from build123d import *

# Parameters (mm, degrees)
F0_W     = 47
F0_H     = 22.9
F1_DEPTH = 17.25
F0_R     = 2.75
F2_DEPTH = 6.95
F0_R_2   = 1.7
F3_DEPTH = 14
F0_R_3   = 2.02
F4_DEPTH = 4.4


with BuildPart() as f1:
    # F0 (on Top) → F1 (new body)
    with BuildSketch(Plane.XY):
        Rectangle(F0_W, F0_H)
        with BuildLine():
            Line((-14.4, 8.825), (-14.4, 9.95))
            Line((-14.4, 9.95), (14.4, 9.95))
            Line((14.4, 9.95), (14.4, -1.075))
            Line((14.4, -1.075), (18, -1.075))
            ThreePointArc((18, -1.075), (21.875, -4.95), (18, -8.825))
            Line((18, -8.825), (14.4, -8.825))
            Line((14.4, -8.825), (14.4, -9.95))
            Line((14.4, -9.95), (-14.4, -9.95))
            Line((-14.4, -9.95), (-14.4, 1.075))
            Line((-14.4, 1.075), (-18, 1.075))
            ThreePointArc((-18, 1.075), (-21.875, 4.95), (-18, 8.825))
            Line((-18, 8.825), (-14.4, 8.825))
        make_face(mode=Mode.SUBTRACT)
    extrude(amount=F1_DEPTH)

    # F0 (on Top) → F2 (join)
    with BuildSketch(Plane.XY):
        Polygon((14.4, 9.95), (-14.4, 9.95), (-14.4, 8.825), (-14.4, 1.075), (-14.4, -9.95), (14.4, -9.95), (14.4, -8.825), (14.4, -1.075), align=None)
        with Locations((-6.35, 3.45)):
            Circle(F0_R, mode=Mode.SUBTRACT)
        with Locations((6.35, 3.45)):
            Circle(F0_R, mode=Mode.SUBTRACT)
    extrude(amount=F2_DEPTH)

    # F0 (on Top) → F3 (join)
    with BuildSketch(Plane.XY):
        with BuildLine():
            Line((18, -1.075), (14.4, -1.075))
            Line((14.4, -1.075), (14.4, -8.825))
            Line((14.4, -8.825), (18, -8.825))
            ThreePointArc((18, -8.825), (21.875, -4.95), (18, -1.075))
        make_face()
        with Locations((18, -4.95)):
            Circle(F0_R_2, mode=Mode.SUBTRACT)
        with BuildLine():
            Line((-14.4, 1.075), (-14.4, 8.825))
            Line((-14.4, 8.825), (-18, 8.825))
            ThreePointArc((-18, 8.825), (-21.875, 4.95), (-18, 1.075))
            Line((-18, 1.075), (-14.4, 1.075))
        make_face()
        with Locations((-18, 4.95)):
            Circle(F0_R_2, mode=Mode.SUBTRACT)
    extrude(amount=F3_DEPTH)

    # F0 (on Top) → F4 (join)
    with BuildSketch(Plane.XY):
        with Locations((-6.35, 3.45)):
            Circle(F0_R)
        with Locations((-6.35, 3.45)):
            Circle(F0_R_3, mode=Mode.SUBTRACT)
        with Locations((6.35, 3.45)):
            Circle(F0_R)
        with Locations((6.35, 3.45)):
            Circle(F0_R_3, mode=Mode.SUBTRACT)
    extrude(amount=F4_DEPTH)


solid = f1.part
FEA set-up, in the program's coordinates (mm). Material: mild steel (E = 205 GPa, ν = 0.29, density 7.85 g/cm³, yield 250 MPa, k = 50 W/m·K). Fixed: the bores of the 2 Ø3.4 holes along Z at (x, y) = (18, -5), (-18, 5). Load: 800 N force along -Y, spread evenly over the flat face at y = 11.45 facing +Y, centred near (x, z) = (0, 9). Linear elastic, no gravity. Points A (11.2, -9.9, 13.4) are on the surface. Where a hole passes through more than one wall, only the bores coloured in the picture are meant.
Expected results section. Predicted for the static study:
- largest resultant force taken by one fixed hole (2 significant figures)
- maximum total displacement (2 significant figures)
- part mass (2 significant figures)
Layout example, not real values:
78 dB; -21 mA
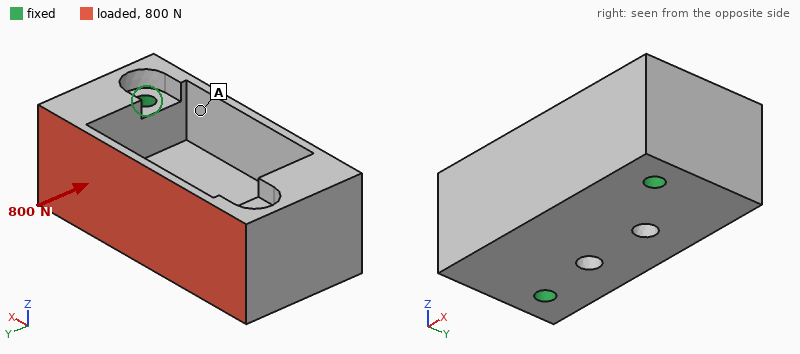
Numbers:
410 N; 17 µm; 93 g
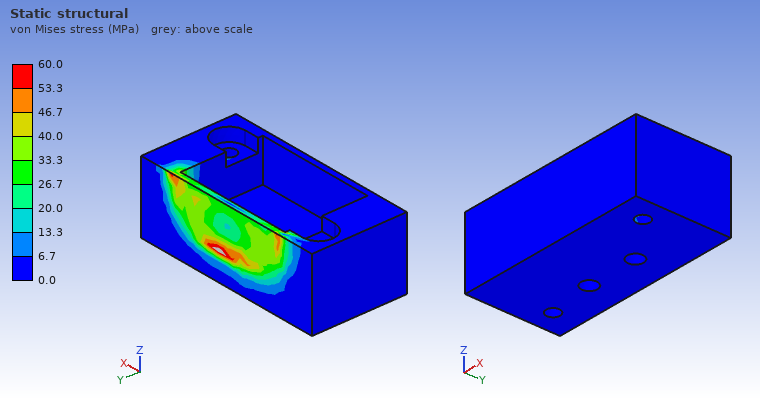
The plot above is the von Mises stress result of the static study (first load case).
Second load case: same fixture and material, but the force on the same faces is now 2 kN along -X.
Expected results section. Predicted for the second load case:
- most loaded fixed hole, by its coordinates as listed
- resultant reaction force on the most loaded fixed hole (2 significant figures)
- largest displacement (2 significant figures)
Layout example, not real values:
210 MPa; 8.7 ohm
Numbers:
(-18, 5); 1.4 kN; 3.0 µm
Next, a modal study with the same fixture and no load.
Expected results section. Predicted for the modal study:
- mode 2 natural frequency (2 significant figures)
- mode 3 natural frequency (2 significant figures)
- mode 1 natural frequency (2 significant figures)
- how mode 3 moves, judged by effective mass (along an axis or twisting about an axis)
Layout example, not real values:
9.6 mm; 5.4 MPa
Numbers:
16 kHz; 22 kHz; 15 kHz; along Z
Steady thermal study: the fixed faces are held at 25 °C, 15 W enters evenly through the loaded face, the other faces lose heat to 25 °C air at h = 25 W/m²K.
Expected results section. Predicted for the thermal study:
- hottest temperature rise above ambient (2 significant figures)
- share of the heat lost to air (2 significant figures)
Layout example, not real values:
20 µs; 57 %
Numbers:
22 K; 3.6 %
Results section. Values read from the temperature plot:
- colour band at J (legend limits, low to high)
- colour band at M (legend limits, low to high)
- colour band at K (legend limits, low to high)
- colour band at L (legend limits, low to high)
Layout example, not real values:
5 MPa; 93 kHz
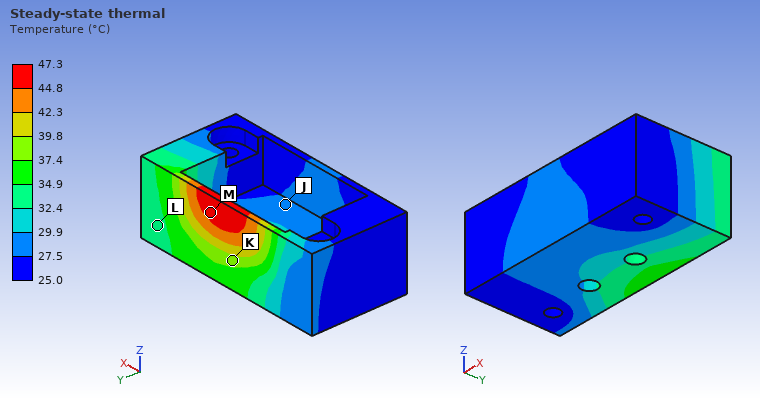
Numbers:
27.5 to 29.9 °C; 44.8 to 47.3 °C; 37.4 to 39.8 °C; 32.4 to 34.9 °C
